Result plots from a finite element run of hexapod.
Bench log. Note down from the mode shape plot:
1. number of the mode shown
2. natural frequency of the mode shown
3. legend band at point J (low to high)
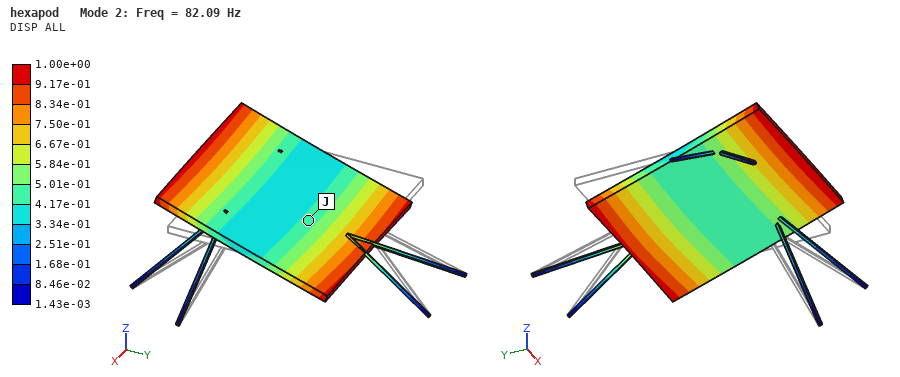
2
82.09 Hz
4.17e-01 to 5.01e-01
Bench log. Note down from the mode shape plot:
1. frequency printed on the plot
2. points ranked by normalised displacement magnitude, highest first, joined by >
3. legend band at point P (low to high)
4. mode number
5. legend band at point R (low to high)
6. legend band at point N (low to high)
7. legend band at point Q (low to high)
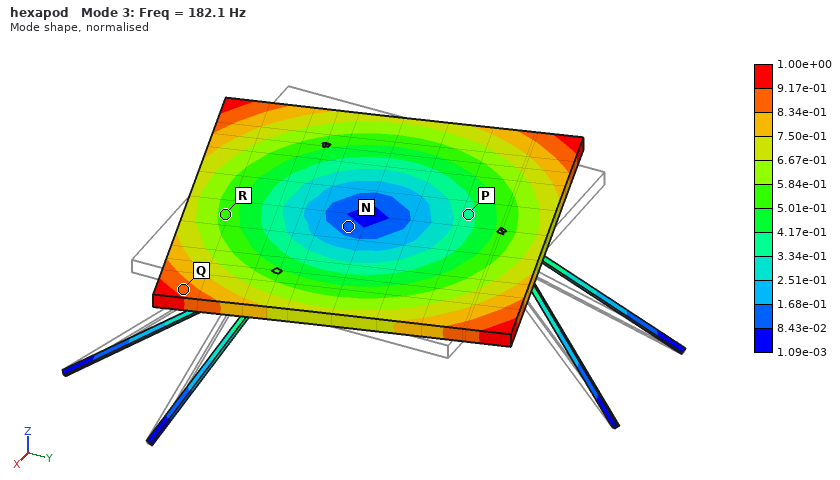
182.1 Hz
Q > R > P > N
3.34e-01 to 4.17e-01
3
5.01e-01 to 5.84e-01
8.43e-02 to 1.68e-01
8.34e-01 to 9.17e-01
